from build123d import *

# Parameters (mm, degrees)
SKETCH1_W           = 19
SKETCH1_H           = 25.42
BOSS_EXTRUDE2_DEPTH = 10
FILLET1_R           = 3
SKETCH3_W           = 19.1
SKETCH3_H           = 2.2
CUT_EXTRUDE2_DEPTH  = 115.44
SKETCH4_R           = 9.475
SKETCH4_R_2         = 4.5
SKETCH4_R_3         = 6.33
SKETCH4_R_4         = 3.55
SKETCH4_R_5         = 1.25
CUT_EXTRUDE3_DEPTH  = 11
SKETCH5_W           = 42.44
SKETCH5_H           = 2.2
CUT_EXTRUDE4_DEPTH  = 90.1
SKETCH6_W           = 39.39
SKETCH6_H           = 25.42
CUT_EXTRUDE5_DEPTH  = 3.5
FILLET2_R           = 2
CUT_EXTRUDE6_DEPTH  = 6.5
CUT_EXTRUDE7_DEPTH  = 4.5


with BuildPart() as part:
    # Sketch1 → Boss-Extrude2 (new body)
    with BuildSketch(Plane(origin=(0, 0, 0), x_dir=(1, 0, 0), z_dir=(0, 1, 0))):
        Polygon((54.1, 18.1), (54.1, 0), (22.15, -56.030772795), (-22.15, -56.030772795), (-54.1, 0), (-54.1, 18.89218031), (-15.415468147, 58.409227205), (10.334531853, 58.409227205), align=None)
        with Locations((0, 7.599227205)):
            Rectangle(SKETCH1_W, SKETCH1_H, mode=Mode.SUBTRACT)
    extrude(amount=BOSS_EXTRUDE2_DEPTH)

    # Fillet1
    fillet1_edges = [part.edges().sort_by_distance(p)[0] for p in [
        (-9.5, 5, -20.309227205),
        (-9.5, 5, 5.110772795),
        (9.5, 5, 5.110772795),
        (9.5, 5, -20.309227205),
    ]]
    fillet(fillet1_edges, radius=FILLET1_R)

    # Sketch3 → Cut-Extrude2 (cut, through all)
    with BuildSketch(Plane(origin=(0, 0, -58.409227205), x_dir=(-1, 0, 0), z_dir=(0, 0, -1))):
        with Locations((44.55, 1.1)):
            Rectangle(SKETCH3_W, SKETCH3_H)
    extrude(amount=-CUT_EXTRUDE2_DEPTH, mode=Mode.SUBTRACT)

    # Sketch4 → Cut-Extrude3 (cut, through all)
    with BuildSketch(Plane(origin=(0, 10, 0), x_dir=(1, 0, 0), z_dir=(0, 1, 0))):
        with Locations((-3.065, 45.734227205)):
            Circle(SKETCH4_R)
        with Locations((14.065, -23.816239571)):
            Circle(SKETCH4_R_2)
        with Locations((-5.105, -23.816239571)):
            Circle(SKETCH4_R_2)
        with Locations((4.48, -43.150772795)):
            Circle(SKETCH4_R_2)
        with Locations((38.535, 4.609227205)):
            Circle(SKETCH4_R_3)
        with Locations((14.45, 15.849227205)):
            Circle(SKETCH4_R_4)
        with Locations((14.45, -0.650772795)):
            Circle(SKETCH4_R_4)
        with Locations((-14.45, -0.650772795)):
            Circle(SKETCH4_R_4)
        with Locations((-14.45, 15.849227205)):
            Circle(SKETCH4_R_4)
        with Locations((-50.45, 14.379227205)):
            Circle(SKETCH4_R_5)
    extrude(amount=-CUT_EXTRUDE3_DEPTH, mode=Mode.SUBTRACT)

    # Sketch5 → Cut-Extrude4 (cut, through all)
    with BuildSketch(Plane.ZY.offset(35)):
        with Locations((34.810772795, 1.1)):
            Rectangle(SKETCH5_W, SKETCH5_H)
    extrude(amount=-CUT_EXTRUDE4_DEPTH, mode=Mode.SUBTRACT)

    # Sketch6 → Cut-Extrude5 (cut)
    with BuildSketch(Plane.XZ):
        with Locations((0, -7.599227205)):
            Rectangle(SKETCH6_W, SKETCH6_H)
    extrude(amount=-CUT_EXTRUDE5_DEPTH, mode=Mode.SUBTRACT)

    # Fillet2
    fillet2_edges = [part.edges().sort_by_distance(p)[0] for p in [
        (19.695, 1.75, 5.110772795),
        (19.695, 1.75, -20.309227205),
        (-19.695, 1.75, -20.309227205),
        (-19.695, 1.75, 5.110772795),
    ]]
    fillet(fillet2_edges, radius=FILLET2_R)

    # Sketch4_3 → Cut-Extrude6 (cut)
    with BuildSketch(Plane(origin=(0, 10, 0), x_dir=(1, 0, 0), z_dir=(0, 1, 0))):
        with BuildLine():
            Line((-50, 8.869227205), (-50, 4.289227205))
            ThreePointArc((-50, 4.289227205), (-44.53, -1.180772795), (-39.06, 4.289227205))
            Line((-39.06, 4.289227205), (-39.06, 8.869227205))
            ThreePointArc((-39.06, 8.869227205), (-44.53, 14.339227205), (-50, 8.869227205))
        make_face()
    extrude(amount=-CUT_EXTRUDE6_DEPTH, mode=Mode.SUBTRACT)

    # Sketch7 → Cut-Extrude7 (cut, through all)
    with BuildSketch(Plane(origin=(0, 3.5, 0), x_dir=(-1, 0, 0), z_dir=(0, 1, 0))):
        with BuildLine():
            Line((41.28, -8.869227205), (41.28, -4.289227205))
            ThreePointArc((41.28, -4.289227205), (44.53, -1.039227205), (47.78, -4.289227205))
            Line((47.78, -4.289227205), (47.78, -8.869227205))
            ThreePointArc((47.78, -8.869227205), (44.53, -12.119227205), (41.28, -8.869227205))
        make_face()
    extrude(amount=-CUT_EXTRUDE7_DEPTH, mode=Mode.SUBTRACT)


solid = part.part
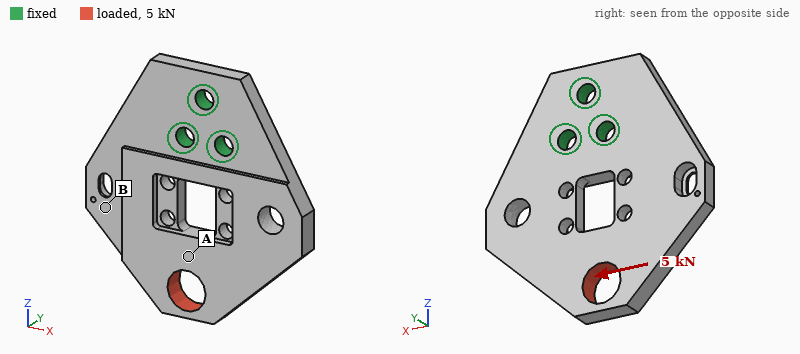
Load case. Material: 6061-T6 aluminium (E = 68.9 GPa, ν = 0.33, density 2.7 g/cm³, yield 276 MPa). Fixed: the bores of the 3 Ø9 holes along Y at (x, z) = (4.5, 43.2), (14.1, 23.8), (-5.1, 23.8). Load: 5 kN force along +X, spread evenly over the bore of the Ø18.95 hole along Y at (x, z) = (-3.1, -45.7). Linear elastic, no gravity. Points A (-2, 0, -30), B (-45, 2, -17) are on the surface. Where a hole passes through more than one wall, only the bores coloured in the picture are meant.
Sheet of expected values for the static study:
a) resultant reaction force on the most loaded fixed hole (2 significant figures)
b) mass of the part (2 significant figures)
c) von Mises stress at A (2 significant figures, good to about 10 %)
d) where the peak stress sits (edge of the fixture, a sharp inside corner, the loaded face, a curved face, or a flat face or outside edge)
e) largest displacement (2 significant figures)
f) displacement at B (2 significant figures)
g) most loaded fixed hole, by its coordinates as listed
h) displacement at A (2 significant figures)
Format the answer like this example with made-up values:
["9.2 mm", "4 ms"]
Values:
["9.3 kN", "180 g", "41 MPa", "a curved face", "0.16 mm", "0.11 mm", "(-5.1, 23.8)", "0.11 mm"]
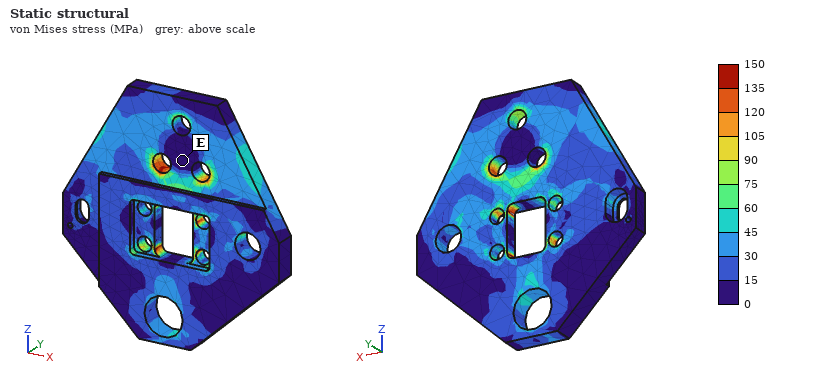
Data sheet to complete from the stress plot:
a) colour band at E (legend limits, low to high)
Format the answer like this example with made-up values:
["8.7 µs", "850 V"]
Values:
["0 to 15 MPa"]
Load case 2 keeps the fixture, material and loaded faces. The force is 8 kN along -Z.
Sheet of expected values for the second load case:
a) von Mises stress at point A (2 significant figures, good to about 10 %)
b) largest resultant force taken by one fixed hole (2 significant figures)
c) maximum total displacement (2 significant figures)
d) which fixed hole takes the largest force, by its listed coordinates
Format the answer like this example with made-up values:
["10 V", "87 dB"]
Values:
["11 MPa", "4.6 kN", "0.10 mm", "(-5.1, 23.8)"]
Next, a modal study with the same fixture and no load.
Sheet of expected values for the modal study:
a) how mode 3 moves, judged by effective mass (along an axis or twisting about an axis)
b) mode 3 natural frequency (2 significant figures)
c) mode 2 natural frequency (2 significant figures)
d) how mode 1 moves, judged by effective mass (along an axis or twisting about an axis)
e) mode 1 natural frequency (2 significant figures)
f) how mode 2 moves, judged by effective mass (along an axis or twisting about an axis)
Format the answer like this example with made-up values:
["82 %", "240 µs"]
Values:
["along X", "3800 Hz", "2000 Hz", "along Y", "1100 Hz", "twisting about Z"]
